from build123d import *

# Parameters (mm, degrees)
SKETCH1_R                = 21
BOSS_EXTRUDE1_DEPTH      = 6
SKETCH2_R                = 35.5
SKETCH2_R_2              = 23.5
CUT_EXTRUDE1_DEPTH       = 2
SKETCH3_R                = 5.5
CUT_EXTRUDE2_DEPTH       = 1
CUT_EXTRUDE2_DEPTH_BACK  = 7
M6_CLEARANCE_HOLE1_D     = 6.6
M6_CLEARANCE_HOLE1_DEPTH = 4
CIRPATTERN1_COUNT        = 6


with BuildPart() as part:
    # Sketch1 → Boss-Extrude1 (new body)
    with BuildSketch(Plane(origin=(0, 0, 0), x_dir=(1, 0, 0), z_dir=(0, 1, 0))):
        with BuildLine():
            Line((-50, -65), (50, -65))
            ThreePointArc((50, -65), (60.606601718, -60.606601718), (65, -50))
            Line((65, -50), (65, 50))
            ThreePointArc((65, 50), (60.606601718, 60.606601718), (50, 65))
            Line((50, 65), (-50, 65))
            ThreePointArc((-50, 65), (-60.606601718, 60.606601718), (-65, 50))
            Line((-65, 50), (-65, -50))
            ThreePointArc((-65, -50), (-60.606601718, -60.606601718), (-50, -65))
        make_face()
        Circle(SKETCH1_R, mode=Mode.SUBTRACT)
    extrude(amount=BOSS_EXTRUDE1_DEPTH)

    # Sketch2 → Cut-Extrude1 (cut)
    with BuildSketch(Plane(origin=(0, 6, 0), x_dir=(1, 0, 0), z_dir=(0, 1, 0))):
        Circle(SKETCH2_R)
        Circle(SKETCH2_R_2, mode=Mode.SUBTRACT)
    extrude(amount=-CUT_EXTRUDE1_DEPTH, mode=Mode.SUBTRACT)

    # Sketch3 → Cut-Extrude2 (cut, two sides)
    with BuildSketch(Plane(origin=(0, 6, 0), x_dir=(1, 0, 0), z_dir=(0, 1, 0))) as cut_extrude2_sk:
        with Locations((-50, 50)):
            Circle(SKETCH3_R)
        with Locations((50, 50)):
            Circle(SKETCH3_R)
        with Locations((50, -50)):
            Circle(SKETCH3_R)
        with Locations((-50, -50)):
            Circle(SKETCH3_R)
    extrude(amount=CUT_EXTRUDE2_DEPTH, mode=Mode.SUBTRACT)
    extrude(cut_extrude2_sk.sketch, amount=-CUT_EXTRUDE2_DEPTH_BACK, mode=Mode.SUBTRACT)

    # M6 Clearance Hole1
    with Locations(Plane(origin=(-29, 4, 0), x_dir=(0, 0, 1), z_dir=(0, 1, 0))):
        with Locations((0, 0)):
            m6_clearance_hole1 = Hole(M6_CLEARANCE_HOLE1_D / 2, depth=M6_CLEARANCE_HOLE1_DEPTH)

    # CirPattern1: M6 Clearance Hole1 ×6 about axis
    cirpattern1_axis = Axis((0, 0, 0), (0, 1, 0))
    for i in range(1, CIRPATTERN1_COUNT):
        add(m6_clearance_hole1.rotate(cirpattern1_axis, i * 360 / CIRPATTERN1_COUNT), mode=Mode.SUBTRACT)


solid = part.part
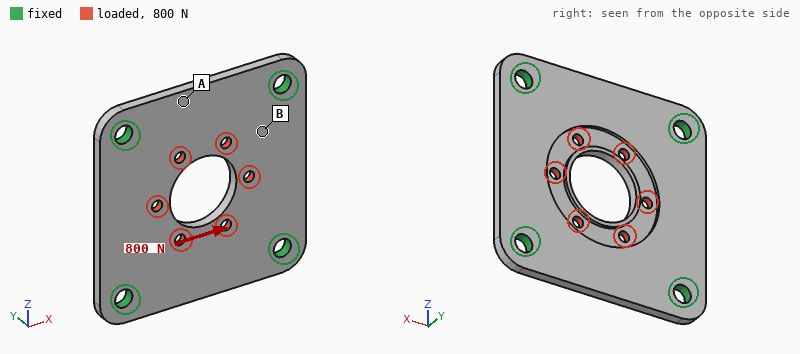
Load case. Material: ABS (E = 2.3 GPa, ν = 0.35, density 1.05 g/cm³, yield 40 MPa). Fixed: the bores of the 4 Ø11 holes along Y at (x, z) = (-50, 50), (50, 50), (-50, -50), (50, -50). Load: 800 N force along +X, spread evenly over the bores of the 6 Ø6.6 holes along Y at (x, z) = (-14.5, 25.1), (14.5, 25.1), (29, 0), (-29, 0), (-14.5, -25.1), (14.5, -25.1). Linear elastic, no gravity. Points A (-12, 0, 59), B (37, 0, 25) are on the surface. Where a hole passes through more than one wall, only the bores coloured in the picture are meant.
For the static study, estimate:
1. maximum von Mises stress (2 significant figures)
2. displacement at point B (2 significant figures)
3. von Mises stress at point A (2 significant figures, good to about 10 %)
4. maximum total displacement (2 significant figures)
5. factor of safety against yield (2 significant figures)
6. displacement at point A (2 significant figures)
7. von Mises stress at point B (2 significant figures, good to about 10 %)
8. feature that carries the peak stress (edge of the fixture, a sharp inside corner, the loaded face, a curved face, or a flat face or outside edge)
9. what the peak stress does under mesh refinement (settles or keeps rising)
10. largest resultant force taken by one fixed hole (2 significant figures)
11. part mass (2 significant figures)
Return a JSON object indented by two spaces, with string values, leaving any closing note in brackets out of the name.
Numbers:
{
  "maximum von Mises stress": "4.0 MPa",
  "displacement at point B": "22 µm",
  "von Mises stress at point A": "0.31 MPa",
  "maximum total displacement": "46 µm",
  "factor of safety against yield": "9.9",
  "displacement at point A": "8.2 µm",
  "von Mises stress at point B": "1.1 MPa",
  "feature that carries the peak stress": "the loaded face",
  "what the peak stress does under mesh refinement": "settles",
  "largest resultant force taken by one fixed hole": "220 N",
  "part mass": "89 g"
}
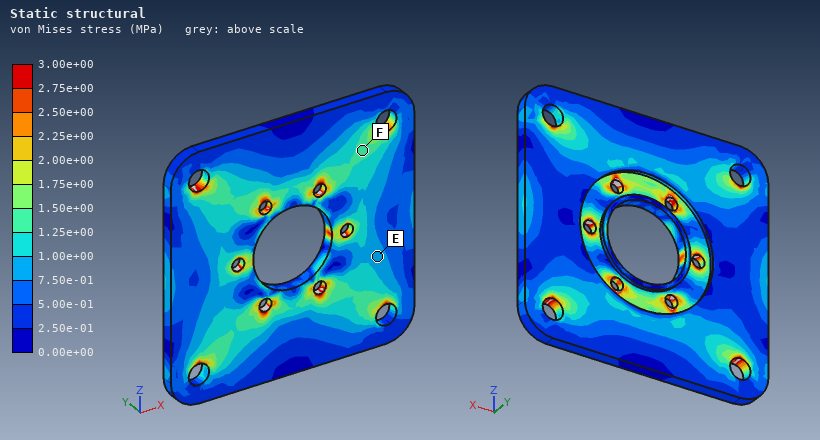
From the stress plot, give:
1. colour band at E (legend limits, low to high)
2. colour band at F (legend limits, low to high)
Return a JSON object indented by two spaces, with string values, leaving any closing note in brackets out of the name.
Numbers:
{
  "colour band at E": "7.50e-01 to 1.00e+00 MPa",
  "colour band at F": "1.25e+00 to 1.50e+00 MPa"
}
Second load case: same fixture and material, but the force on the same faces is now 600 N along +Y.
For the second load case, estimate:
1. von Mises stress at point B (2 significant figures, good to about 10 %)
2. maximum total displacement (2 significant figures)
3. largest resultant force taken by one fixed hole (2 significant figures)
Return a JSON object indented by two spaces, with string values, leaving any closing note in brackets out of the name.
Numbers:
{
  "von Mises stress at point B": "4.8 MPa",
  "maximum total displacement": "1.5 mm",
  "largest resultant force taken by one fixed hole": "170 N"
}
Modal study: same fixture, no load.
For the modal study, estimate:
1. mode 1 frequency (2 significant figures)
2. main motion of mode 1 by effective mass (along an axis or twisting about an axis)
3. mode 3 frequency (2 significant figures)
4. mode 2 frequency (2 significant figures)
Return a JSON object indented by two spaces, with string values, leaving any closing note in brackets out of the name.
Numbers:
{
  "mode 1 frequency": "780 Hz",
  "main motion of mode 1 by effective mass": "along Y",
  "mode 3 frequency": "1000 Hz",
  "mode 2 frequency": "1000 Hz"
}
